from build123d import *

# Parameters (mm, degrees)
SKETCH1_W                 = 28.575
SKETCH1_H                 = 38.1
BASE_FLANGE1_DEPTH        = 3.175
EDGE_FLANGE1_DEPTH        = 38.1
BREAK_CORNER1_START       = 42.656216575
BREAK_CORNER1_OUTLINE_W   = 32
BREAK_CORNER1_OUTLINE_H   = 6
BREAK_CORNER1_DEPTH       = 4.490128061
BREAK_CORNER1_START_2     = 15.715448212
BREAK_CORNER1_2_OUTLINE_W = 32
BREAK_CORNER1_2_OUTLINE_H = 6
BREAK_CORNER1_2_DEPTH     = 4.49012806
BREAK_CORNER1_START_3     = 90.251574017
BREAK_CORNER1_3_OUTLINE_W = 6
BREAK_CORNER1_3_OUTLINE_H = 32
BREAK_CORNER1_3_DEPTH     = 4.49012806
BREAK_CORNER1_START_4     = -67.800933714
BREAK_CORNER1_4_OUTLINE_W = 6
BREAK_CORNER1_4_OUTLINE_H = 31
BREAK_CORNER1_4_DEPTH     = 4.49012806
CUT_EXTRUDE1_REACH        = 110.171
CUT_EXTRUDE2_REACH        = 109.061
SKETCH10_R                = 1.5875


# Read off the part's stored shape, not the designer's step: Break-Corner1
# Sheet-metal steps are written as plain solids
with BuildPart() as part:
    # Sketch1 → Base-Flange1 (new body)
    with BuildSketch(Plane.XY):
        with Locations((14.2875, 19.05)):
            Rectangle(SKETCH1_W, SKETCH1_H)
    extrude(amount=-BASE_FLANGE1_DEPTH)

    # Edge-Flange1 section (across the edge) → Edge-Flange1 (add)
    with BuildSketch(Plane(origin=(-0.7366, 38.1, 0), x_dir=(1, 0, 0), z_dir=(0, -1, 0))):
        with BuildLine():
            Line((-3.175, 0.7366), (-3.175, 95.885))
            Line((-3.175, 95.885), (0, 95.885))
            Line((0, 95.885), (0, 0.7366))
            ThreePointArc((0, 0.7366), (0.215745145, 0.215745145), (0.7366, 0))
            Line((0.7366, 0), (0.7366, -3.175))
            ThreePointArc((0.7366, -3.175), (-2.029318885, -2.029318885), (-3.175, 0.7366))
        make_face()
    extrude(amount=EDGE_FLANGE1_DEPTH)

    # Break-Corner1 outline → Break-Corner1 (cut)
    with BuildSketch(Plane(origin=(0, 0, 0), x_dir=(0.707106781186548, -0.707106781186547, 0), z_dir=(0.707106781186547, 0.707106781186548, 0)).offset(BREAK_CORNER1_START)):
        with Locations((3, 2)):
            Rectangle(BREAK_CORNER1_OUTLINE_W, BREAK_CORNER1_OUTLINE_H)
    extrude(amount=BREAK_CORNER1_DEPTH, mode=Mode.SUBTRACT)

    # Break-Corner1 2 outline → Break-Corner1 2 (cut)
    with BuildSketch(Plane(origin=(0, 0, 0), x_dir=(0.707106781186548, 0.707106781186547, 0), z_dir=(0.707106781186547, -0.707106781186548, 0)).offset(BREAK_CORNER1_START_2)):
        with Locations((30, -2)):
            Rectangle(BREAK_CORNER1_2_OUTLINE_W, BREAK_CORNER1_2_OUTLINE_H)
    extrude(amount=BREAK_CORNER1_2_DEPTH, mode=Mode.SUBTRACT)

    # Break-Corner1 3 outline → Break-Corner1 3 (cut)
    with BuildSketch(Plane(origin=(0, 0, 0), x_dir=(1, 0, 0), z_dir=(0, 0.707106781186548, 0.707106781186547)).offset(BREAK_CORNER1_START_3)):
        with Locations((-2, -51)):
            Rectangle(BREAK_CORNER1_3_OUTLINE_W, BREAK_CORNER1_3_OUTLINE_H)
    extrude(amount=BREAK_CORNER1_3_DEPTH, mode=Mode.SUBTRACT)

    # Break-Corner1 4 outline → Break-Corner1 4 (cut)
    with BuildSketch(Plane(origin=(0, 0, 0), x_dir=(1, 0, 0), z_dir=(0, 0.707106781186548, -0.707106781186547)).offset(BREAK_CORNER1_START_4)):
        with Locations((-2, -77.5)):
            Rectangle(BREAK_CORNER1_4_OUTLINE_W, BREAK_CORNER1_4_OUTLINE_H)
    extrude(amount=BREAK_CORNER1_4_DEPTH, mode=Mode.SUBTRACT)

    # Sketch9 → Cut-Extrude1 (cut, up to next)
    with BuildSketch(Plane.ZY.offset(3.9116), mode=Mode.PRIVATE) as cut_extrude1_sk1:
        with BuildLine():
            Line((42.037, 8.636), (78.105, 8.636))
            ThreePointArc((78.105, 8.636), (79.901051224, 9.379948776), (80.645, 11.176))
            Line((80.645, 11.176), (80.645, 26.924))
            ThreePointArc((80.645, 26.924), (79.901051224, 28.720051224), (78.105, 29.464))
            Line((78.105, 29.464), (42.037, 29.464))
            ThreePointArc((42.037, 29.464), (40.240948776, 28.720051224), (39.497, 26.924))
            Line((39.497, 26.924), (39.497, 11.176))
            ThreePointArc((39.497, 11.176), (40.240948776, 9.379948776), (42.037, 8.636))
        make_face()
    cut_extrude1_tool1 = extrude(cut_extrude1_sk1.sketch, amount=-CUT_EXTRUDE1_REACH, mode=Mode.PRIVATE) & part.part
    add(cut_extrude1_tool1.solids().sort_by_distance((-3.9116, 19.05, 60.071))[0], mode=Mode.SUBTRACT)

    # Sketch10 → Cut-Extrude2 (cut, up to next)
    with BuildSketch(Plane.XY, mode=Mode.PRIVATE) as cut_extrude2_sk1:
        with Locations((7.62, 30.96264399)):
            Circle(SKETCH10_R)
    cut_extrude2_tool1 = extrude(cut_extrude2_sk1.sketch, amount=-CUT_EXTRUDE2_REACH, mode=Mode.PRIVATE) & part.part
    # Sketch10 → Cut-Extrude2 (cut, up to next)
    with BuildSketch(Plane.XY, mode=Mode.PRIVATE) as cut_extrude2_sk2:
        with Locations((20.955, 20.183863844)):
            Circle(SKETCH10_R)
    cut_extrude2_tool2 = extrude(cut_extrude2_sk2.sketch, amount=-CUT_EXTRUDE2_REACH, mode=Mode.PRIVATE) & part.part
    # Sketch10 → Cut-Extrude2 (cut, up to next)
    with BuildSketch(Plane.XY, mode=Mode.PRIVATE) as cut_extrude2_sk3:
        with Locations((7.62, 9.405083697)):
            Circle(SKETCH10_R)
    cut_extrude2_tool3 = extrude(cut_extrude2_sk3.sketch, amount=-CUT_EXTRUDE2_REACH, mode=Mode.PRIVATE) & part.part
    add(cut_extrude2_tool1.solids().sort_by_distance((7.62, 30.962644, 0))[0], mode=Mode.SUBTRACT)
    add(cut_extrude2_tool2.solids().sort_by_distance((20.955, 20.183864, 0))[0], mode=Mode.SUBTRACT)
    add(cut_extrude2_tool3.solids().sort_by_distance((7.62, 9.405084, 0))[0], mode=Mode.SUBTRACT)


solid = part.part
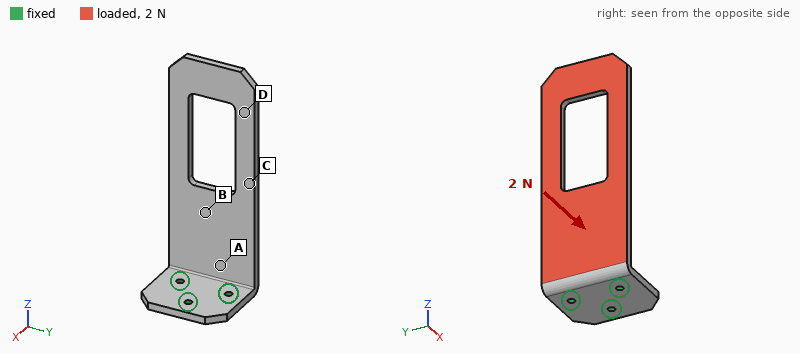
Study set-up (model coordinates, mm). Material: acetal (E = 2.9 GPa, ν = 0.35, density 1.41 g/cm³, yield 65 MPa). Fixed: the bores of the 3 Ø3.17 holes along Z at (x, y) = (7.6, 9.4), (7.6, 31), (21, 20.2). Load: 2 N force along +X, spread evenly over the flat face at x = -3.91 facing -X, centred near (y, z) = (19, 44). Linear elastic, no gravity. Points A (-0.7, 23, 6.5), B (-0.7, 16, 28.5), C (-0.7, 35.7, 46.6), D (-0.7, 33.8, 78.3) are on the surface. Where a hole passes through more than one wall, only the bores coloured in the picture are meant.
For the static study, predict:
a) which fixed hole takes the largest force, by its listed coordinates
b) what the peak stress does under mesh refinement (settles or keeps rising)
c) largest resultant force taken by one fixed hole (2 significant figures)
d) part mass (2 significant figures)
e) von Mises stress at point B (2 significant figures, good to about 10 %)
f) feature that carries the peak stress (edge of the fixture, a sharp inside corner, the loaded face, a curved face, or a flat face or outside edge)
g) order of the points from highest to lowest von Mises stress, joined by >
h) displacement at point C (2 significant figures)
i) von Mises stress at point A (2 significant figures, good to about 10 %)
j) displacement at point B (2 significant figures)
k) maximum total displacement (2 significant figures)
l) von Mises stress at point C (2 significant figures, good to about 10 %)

(21, 20.2)
keeps rising
1.8 N
17 g
0.56 MPa
edge of the fixture
A > C > B > D
0.37 mm
1.1 MPa
0.19 mm
1.1 mm
0.81 MPa
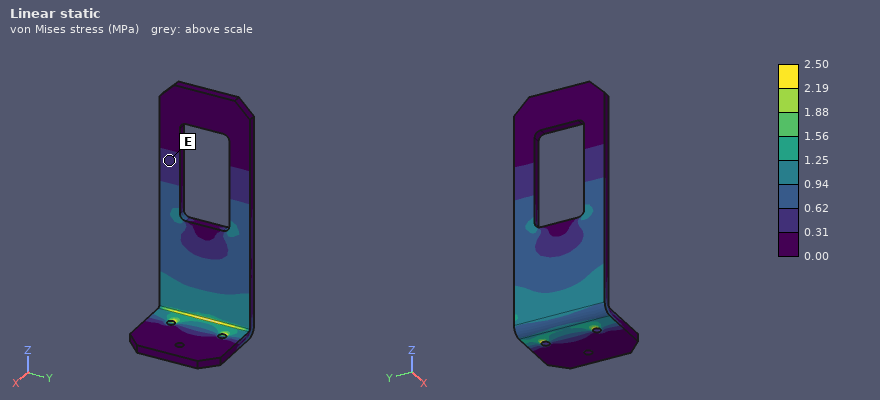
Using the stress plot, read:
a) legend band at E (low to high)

0.31 to 0.62 MPa
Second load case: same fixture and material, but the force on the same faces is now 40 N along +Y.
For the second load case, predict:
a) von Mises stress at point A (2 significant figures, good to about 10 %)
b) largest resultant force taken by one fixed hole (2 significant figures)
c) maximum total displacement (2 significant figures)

3.3 MPa
82 N
1.2 mm
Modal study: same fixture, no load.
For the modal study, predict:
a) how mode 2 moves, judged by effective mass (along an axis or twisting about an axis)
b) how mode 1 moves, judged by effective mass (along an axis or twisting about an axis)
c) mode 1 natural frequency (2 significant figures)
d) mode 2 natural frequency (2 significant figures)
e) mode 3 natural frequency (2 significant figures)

along Y
along X
76 Hz
300 Hz
370 Hz
